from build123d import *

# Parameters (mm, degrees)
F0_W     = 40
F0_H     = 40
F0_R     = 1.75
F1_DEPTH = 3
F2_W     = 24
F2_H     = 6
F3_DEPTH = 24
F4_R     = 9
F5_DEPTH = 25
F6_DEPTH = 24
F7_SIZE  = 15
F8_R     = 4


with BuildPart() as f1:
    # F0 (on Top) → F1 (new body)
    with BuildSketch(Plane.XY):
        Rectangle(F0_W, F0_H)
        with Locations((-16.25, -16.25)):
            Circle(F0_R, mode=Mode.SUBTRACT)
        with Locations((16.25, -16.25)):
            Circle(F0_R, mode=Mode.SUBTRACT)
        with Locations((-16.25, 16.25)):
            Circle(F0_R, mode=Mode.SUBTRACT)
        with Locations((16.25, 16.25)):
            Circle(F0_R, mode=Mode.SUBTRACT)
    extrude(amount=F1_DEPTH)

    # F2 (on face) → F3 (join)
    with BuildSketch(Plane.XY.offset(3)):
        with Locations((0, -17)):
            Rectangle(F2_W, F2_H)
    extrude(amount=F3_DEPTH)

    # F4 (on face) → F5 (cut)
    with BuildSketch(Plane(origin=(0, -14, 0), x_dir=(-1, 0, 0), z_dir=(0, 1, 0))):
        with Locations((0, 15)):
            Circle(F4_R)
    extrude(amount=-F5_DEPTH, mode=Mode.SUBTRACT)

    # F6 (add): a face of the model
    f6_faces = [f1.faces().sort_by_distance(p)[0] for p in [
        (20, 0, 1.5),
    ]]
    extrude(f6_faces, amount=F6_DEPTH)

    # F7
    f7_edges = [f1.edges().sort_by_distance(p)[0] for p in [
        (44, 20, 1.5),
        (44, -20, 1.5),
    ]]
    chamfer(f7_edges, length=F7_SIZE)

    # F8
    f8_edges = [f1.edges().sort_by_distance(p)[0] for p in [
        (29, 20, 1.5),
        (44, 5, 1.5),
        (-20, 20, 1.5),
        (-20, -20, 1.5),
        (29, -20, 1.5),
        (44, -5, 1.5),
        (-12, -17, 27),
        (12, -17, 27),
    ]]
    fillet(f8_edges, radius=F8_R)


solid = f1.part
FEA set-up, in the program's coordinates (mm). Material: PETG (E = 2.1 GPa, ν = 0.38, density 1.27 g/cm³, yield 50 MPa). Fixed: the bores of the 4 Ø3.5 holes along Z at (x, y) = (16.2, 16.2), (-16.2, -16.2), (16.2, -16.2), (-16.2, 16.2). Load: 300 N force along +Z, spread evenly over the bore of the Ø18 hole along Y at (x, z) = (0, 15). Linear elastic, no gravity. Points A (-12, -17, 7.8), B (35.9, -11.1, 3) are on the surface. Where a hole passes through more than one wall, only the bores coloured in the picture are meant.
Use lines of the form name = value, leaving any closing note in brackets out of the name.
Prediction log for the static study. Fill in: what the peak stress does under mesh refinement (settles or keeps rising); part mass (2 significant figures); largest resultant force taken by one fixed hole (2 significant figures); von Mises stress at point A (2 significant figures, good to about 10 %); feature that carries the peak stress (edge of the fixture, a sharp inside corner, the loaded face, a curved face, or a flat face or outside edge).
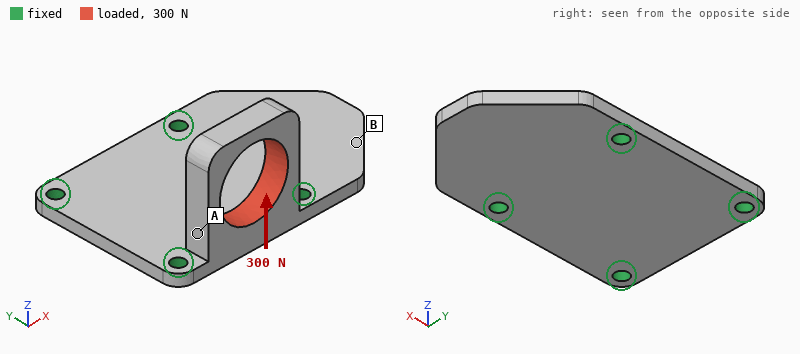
what the peak stress does under mesh refinement = keeps rising
part mass = 11 g
largest resultant force taken by one fixed hole = 160 N
von Mises stress at point A = 9.7 MPa
feature that carries the peak stress = edge of the fixture
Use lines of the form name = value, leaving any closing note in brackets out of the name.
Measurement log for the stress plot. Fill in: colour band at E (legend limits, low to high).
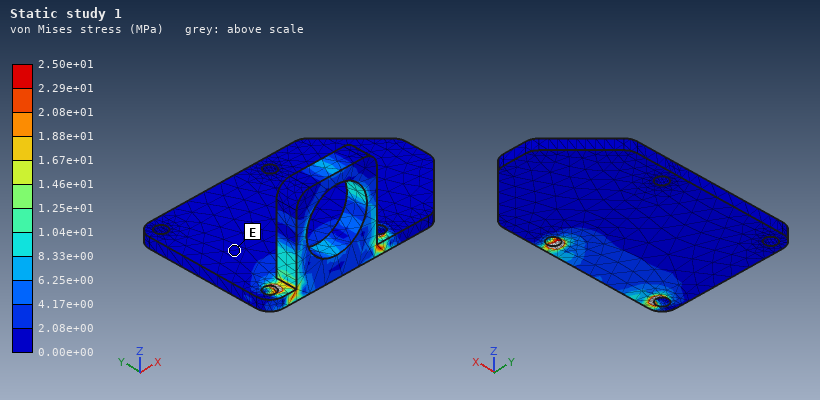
colour band at E = 0.00e+00 to 2.08e+00 MPa
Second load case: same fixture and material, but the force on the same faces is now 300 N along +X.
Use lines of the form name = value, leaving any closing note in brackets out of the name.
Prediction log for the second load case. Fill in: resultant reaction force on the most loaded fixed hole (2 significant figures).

resultant reaction force on the most loaded fixed hole = 210 N
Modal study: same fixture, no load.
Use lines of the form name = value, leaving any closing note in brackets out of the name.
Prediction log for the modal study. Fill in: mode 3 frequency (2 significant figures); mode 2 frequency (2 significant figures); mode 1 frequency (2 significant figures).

mode 3 frequency = 2300 Hz
mode 2 frequency = 1100 Hz
mode 1 frequency = 980 Hz
